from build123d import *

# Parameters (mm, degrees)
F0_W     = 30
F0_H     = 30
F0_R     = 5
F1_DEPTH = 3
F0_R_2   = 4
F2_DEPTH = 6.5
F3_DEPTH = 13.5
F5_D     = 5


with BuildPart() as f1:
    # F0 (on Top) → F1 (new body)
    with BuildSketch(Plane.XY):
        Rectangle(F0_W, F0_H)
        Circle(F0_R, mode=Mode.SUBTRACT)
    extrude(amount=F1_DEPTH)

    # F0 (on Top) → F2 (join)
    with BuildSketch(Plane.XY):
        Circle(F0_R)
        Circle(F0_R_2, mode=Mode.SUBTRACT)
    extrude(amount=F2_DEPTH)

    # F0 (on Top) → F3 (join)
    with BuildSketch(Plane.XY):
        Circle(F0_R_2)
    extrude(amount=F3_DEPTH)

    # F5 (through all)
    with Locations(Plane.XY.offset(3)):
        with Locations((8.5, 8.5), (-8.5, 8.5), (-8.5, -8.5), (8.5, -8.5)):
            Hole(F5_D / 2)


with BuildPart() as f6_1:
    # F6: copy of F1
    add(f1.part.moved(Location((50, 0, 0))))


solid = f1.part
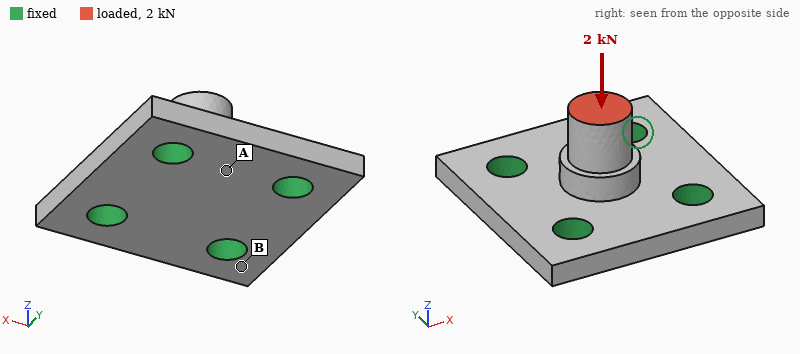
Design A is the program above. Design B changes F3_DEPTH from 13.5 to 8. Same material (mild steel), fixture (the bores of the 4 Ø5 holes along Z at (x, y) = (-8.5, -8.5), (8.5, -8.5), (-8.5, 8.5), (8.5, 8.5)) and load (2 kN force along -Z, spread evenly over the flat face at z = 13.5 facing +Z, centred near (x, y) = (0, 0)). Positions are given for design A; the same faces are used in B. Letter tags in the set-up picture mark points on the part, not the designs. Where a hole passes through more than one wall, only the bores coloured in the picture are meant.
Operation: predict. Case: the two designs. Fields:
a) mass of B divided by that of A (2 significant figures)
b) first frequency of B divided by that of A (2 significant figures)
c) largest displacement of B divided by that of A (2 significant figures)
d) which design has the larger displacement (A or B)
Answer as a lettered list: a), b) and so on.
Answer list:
a) 0.91
b) 1.4
c) 0.85
d) A
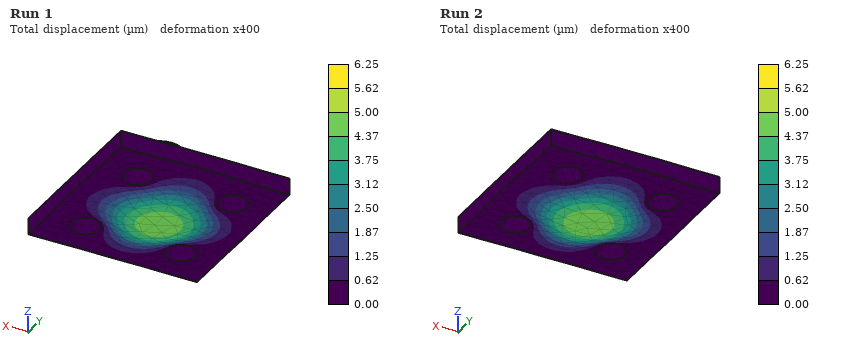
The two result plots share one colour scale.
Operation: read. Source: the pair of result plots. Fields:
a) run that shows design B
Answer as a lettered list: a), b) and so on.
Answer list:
a) Run 2
